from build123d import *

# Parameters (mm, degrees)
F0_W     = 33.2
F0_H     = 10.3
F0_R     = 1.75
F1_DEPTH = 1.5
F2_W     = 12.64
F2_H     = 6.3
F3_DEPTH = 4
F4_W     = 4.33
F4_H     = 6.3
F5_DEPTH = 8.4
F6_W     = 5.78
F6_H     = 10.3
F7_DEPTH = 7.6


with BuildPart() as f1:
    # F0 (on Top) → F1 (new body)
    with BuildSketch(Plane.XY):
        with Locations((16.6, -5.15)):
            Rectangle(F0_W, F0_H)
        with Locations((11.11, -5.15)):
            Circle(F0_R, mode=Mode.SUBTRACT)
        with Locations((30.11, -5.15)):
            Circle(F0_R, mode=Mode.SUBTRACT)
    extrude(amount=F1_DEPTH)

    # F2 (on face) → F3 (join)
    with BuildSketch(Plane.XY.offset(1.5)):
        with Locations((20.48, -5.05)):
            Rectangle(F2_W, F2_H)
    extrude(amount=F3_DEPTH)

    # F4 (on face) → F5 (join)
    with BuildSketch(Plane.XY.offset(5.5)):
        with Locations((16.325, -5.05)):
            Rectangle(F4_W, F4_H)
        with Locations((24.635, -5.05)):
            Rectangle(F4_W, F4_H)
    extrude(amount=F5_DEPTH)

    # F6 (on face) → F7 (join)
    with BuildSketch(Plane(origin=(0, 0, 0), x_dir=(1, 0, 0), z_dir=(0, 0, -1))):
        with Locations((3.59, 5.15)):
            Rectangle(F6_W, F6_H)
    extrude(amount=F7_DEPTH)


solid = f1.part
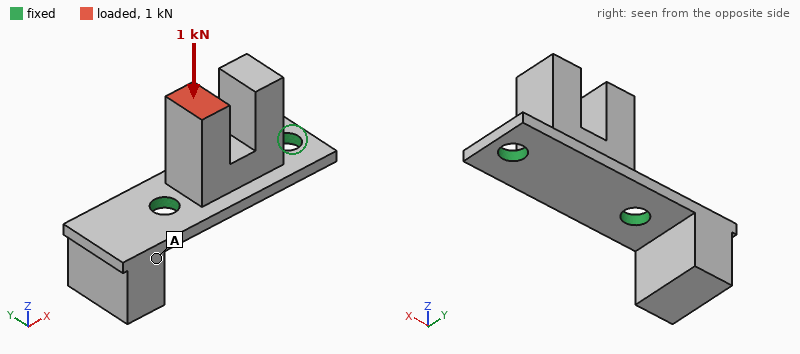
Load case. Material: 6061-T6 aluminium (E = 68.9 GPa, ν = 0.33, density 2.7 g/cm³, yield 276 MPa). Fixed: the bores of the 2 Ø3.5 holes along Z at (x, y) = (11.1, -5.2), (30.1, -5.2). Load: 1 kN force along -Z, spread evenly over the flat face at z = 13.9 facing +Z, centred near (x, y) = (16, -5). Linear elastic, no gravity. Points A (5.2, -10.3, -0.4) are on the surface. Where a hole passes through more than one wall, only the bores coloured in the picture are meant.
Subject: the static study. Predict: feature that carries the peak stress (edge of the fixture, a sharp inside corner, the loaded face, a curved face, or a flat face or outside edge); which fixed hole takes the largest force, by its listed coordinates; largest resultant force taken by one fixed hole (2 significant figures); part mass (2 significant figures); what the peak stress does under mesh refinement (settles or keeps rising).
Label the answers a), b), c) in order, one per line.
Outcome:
a) edge of the fixture
b) (11.1, -5.2)
c) 840 N
d) 4.6 g
e) keeps rising
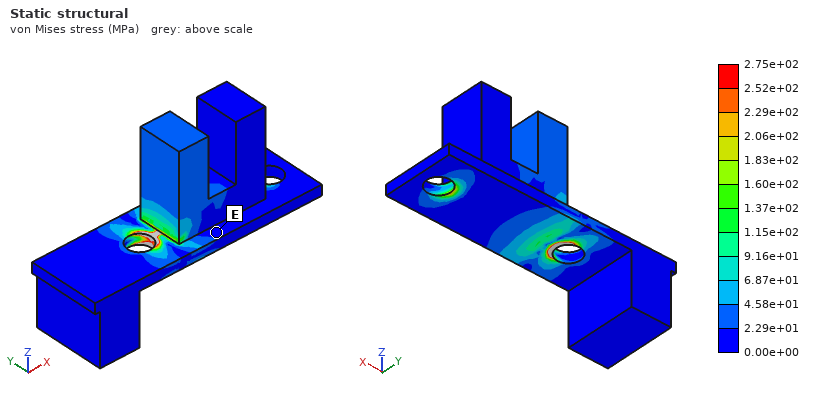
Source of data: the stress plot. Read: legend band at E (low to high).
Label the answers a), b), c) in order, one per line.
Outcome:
a) 0.00e+00 to 2.29e+01 MPa
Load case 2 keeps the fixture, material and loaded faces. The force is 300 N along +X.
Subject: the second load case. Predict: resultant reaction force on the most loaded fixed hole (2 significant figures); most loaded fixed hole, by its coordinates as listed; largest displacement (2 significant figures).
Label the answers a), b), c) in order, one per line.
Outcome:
a) 400 N
b) (30.1, -5.2)
c) 62 µm
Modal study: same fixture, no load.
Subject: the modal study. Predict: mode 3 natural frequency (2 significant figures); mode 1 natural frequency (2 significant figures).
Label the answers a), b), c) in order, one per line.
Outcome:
a) 8200 Hz
b) 4300 Hz
